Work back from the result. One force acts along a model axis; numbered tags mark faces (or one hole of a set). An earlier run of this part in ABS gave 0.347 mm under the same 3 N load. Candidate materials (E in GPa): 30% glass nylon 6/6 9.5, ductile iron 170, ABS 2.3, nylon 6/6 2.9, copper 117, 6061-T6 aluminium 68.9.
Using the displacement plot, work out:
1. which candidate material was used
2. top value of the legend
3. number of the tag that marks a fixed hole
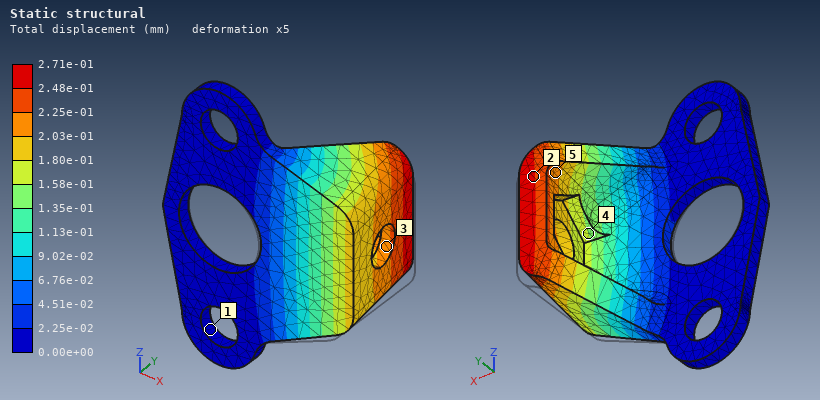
nylon 6/6
2.71e-01 mm
1
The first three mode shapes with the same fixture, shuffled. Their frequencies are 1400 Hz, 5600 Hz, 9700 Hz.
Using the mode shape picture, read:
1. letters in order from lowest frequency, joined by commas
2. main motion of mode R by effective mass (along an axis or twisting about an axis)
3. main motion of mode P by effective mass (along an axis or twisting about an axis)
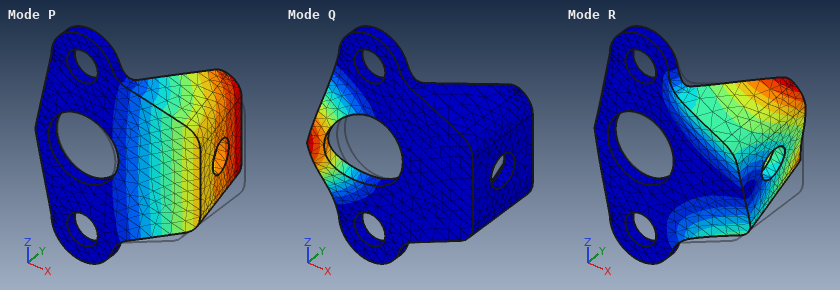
P, R, Q
along Z
along Y
